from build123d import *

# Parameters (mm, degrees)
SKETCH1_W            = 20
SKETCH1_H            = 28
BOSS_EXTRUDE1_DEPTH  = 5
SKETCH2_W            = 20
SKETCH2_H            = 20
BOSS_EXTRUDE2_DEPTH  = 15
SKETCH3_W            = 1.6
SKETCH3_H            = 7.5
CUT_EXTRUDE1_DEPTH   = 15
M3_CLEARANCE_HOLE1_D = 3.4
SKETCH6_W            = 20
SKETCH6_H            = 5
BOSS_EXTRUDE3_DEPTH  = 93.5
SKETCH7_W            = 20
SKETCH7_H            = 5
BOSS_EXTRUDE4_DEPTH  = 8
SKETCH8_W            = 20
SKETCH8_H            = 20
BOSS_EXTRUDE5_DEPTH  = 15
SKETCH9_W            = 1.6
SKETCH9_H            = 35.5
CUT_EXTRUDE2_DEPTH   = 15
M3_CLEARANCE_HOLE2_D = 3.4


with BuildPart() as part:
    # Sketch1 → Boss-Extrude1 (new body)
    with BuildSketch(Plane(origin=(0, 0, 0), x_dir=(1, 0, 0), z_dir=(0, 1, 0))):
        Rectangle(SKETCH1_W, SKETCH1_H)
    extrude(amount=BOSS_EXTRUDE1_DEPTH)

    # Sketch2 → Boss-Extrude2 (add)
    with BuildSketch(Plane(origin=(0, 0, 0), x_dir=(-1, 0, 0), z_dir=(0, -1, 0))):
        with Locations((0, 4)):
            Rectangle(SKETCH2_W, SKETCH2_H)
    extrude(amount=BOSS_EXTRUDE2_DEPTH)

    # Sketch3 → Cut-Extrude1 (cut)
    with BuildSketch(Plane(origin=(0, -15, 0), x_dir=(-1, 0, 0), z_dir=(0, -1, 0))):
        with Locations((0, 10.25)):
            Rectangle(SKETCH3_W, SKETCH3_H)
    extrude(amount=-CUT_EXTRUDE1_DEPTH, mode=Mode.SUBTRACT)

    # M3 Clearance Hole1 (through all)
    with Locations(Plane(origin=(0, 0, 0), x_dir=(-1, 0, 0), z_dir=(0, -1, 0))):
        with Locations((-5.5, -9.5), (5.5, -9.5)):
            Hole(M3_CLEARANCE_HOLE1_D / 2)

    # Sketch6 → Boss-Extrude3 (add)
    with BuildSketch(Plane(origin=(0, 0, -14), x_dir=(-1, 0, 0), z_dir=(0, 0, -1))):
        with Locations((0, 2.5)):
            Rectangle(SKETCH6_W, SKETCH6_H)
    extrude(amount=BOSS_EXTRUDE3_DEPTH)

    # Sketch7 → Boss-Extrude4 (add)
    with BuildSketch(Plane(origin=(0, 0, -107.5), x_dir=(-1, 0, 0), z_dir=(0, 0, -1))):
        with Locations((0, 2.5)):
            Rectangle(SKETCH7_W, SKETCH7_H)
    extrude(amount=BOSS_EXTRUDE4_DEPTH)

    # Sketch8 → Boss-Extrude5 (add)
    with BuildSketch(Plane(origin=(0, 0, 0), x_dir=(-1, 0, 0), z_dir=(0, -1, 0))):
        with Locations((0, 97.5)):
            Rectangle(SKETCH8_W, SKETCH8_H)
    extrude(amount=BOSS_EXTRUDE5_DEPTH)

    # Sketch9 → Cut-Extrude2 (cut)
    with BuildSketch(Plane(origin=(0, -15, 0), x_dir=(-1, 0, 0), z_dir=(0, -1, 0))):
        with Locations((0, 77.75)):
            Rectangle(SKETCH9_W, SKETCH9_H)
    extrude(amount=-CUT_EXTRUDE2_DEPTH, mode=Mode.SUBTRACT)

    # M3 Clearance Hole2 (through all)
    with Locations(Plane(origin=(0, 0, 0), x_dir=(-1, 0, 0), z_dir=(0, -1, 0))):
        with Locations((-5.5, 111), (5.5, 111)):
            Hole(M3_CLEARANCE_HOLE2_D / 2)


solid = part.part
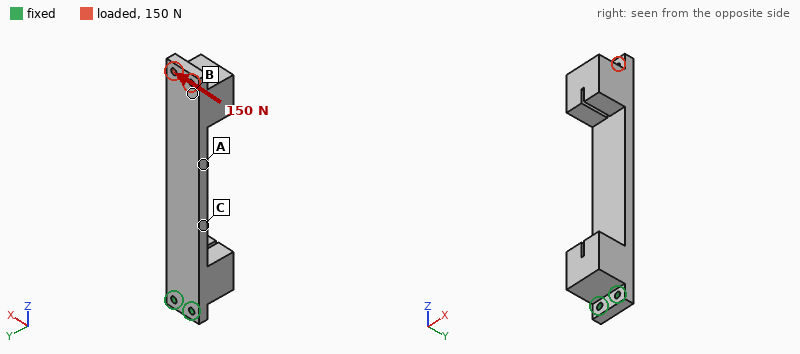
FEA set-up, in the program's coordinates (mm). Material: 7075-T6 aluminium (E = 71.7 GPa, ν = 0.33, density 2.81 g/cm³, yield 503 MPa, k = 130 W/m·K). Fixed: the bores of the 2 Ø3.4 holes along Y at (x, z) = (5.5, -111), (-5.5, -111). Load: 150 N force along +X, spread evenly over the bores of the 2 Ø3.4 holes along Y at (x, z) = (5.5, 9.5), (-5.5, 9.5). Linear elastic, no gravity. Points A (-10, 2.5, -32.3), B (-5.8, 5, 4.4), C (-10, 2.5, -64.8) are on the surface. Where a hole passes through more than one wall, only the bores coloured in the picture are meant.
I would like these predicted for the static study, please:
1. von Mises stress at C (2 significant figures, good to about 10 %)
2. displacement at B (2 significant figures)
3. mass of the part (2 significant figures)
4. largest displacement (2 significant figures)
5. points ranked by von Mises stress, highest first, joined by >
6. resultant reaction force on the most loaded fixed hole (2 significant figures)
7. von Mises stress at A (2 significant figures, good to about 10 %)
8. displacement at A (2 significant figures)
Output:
33 MPa
0.32 mm
69 g
0.36 mm
C > A > B
1.4 kN
19 MPa
0.17 mm
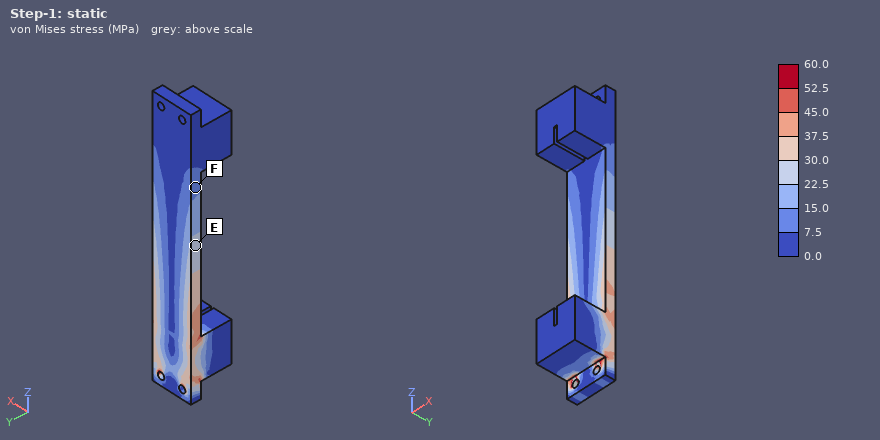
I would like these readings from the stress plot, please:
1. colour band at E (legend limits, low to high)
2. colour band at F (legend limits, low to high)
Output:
22.5 to 30.0 MPa
7.5 to 15.0 MPa
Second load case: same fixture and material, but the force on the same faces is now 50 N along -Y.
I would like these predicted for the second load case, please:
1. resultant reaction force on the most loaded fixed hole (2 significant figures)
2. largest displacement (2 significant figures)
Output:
25 N
1.4 mm
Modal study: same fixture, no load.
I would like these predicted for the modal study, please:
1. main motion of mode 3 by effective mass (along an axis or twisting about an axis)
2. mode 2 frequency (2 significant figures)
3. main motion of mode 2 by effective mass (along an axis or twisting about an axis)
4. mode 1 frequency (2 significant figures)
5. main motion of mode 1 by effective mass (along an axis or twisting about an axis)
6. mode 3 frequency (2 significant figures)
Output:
along Y
700 Hz
along X
220 Hz
along Y
1500 Hz
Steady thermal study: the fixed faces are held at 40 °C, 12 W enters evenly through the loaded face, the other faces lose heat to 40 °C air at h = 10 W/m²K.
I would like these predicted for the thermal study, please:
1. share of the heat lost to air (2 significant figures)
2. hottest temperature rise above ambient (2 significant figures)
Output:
28 %
76 K
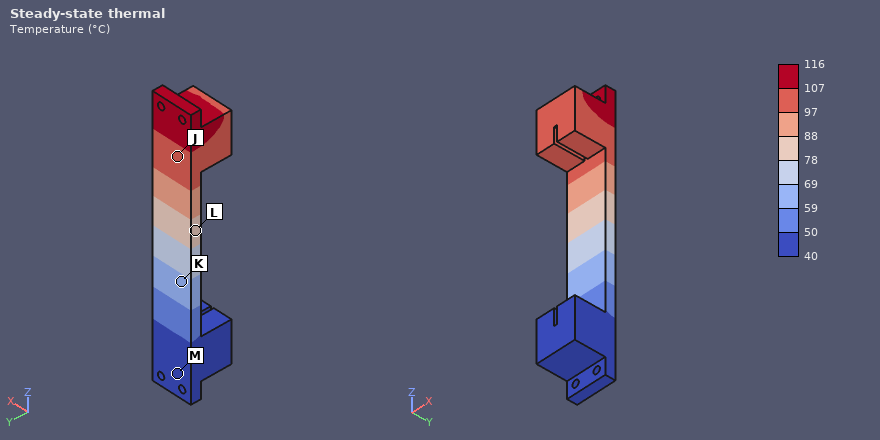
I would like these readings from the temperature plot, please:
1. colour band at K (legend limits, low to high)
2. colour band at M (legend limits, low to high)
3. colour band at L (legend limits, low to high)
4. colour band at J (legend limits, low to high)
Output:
59 to 69 °C
40 to 50 °C
78 to 88 °C
97 to 107 °C
